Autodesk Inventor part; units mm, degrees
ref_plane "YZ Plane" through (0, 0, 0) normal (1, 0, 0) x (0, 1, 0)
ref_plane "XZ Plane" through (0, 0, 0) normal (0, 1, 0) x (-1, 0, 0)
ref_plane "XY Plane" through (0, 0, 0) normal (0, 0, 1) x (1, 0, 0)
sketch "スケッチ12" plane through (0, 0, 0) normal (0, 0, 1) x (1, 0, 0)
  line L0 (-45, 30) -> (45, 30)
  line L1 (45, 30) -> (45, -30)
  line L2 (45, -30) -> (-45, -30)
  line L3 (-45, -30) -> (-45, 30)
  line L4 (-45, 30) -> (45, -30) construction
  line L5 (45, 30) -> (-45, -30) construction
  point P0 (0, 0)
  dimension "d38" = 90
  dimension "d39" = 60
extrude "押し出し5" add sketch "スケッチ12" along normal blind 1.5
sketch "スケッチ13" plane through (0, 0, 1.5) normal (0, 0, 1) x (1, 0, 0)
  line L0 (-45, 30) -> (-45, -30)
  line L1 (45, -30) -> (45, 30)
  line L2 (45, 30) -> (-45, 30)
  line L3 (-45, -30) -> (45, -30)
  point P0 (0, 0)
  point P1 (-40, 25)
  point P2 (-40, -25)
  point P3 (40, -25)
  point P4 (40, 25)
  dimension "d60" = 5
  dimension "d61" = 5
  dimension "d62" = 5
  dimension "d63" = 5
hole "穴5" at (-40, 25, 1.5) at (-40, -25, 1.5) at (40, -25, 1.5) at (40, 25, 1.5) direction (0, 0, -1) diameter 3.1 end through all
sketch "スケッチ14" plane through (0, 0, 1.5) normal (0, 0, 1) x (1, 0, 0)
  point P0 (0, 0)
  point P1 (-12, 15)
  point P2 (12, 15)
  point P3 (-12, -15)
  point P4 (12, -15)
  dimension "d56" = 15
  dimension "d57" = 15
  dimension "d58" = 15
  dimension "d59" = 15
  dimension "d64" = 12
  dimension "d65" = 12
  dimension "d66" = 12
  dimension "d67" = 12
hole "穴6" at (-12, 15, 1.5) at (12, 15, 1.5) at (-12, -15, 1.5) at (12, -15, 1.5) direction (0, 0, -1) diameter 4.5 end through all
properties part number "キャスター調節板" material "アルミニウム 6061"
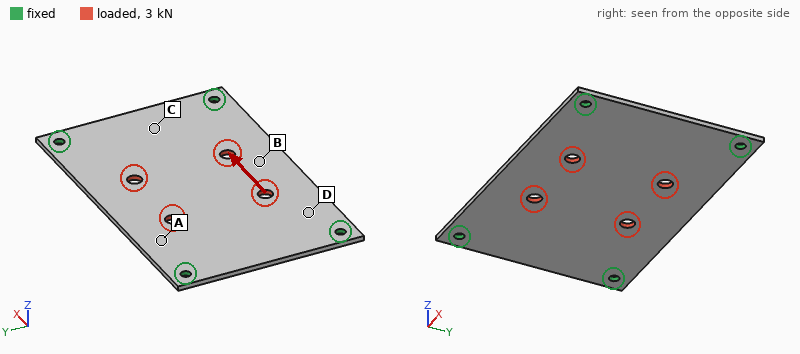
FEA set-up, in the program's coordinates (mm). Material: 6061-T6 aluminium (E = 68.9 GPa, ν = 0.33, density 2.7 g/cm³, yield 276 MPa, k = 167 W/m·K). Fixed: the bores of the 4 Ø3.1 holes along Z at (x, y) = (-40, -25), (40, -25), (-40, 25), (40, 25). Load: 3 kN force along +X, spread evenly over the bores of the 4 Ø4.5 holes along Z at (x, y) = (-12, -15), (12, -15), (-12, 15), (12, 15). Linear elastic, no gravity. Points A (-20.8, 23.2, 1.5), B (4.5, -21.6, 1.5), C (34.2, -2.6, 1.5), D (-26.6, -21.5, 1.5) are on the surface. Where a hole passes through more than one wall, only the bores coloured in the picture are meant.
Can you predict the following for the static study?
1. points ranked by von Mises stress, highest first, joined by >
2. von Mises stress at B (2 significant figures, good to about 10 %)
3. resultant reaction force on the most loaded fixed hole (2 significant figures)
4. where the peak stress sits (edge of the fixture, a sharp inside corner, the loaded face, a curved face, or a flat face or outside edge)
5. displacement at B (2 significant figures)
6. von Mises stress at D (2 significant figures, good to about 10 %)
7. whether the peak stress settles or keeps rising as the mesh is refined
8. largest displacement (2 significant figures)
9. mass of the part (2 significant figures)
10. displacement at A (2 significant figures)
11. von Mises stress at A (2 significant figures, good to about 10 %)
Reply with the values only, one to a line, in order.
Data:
D > A > B > C
14 MPa
780 N
edge of the fixture
13 µm
29 MPa
keeps rising
17 µm
21 g
9.8 µm
24 MPa
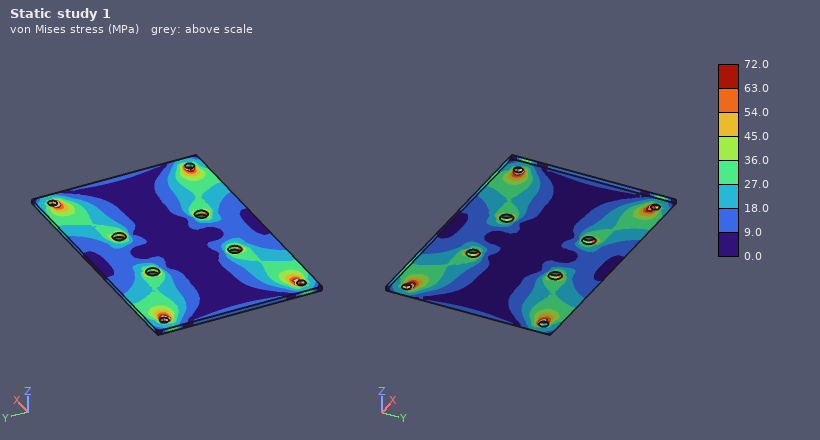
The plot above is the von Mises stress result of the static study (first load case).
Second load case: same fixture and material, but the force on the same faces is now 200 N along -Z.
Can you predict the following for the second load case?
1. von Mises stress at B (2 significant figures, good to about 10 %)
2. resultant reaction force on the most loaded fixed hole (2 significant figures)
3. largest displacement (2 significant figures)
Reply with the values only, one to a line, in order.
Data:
49 MPa
50 N
0.50 mm
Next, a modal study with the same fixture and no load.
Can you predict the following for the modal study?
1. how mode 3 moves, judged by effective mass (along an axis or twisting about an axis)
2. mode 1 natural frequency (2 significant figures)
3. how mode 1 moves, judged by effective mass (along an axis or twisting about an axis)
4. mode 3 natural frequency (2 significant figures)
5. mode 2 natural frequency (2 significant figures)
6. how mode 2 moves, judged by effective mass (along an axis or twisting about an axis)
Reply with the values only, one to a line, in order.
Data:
twisting about Y
1000 Hz
along Z
2600 Hz
1600 Hz
twisting about X
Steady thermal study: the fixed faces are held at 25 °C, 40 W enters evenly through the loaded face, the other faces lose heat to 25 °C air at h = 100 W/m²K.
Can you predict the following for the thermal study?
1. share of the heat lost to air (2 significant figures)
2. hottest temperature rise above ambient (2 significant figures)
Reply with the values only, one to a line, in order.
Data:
52 %
37 K
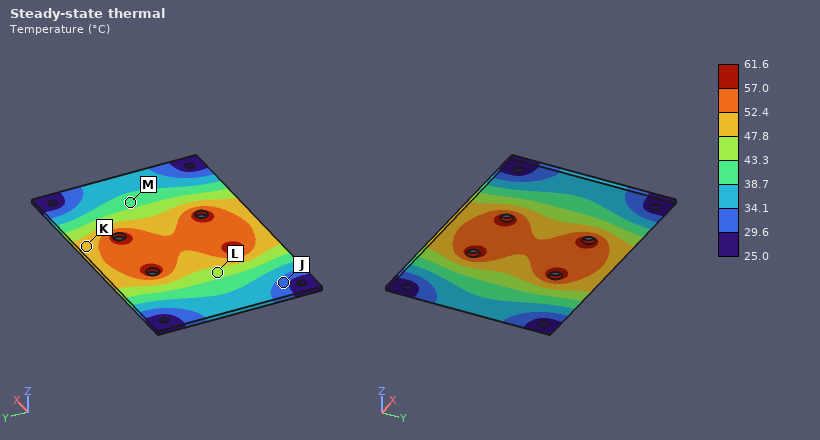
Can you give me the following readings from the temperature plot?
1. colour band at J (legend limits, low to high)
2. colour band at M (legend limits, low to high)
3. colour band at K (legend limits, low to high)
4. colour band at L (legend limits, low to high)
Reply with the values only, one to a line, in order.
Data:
29.6 to 34.1 °C
38.7 to 43.3 °C
47.8 to 52.4 °C
43.3 to 47.8 °C
